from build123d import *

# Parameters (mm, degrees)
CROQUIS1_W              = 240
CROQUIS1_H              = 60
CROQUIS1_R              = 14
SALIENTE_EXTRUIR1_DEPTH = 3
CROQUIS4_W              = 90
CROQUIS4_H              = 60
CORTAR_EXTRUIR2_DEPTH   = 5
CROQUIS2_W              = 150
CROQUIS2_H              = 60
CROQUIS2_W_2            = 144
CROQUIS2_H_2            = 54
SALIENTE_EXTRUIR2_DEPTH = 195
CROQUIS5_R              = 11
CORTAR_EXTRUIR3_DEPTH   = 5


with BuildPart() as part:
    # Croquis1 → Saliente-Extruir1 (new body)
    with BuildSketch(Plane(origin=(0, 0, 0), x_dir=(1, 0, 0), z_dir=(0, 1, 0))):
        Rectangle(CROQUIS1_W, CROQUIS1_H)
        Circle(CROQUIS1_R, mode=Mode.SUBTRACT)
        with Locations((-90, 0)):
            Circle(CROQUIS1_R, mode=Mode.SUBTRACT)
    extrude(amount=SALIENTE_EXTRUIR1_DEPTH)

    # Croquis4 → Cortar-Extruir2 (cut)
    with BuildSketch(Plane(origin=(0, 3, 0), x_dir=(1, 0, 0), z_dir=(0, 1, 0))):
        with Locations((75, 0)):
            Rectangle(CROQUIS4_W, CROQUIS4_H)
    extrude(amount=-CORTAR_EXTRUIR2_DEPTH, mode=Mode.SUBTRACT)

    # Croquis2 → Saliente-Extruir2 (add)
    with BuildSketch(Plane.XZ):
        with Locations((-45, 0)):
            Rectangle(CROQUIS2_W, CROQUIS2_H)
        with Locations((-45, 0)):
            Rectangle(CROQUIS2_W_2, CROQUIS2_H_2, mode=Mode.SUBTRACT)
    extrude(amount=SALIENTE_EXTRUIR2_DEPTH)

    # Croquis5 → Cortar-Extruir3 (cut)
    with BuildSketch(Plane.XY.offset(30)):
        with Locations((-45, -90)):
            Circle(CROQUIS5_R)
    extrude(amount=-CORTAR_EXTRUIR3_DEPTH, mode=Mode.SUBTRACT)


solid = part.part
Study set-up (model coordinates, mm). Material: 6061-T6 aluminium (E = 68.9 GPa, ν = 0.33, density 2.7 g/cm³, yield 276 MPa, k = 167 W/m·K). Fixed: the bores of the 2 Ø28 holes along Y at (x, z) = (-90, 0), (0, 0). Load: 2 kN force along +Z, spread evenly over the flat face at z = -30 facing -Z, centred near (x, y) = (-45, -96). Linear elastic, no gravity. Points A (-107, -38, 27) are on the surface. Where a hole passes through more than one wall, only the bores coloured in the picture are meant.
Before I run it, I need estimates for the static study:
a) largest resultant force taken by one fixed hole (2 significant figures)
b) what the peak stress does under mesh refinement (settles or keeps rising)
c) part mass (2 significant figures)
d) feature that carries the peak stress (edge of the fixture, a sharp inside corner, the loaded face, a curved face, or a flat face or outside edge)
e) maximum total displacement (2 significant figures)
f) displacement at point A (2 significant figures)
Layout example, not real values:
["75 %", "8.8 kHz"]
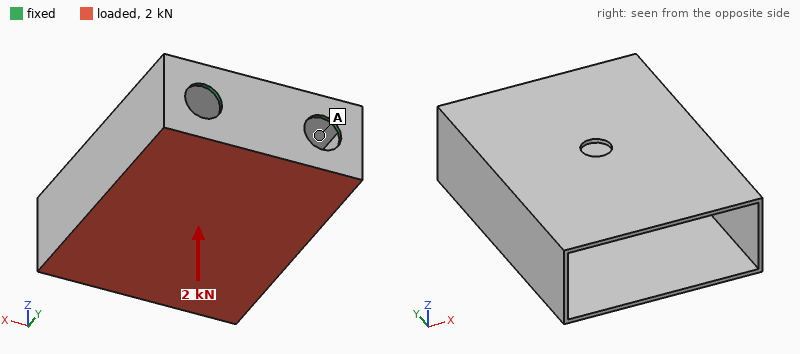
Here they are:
["1.0 kN", "keeps rising", "700 g", "edge of the fixture", "2.7 mm", "0.43 mm"]
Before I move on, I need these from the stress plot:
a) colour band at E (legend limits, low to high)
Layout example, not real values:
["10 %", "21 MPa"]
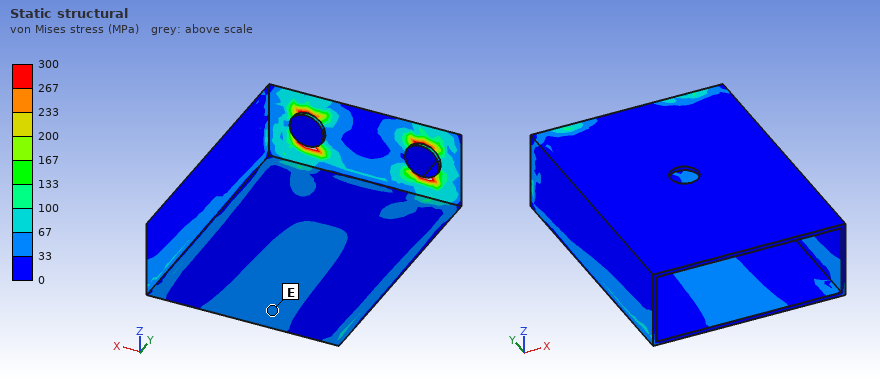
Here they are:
["33 to 67 MPa"]
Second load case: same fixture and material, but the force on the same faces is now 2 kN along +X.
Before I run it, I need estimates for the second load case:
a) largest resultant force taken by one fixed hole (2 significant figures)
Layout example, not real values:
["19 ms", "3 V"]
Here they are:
["2.1 kN"]
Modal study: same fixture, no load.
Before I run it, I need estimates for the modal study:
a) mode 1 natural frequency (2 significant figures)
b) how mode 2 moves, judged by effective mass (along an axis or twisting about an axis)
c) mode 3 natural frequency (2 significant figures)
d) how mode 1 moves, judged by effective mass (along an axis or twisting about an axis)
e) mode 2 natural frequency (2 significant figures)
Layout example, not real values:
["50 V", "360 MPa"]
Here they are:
["240 Hz", "twisting about Y", "550 Hz", "along Z", "430 Hz"]
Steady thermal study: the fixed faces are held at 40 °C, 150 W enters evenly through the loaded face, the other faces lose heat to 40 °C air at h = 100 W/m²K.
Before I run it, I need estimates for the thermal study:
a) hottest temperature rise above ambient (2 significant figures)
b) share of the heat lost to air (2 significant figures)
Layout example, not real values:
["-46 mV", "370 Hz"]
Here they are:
["28 K", "80 %"]
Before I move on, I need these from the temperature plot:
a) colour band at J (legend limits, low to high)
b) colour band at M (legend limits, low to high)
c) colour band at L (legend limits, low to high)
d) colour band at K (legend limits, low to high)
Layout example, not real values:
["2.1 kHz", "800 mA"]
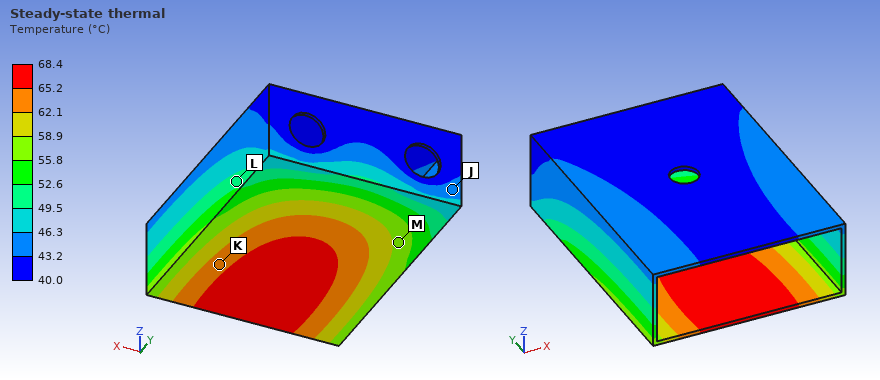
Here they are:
["43.2 to 46.3 °C", "55.8 to 58.9 °C", "49.5 to 52.6 °C", "62.1 to 65.2 °C"]
